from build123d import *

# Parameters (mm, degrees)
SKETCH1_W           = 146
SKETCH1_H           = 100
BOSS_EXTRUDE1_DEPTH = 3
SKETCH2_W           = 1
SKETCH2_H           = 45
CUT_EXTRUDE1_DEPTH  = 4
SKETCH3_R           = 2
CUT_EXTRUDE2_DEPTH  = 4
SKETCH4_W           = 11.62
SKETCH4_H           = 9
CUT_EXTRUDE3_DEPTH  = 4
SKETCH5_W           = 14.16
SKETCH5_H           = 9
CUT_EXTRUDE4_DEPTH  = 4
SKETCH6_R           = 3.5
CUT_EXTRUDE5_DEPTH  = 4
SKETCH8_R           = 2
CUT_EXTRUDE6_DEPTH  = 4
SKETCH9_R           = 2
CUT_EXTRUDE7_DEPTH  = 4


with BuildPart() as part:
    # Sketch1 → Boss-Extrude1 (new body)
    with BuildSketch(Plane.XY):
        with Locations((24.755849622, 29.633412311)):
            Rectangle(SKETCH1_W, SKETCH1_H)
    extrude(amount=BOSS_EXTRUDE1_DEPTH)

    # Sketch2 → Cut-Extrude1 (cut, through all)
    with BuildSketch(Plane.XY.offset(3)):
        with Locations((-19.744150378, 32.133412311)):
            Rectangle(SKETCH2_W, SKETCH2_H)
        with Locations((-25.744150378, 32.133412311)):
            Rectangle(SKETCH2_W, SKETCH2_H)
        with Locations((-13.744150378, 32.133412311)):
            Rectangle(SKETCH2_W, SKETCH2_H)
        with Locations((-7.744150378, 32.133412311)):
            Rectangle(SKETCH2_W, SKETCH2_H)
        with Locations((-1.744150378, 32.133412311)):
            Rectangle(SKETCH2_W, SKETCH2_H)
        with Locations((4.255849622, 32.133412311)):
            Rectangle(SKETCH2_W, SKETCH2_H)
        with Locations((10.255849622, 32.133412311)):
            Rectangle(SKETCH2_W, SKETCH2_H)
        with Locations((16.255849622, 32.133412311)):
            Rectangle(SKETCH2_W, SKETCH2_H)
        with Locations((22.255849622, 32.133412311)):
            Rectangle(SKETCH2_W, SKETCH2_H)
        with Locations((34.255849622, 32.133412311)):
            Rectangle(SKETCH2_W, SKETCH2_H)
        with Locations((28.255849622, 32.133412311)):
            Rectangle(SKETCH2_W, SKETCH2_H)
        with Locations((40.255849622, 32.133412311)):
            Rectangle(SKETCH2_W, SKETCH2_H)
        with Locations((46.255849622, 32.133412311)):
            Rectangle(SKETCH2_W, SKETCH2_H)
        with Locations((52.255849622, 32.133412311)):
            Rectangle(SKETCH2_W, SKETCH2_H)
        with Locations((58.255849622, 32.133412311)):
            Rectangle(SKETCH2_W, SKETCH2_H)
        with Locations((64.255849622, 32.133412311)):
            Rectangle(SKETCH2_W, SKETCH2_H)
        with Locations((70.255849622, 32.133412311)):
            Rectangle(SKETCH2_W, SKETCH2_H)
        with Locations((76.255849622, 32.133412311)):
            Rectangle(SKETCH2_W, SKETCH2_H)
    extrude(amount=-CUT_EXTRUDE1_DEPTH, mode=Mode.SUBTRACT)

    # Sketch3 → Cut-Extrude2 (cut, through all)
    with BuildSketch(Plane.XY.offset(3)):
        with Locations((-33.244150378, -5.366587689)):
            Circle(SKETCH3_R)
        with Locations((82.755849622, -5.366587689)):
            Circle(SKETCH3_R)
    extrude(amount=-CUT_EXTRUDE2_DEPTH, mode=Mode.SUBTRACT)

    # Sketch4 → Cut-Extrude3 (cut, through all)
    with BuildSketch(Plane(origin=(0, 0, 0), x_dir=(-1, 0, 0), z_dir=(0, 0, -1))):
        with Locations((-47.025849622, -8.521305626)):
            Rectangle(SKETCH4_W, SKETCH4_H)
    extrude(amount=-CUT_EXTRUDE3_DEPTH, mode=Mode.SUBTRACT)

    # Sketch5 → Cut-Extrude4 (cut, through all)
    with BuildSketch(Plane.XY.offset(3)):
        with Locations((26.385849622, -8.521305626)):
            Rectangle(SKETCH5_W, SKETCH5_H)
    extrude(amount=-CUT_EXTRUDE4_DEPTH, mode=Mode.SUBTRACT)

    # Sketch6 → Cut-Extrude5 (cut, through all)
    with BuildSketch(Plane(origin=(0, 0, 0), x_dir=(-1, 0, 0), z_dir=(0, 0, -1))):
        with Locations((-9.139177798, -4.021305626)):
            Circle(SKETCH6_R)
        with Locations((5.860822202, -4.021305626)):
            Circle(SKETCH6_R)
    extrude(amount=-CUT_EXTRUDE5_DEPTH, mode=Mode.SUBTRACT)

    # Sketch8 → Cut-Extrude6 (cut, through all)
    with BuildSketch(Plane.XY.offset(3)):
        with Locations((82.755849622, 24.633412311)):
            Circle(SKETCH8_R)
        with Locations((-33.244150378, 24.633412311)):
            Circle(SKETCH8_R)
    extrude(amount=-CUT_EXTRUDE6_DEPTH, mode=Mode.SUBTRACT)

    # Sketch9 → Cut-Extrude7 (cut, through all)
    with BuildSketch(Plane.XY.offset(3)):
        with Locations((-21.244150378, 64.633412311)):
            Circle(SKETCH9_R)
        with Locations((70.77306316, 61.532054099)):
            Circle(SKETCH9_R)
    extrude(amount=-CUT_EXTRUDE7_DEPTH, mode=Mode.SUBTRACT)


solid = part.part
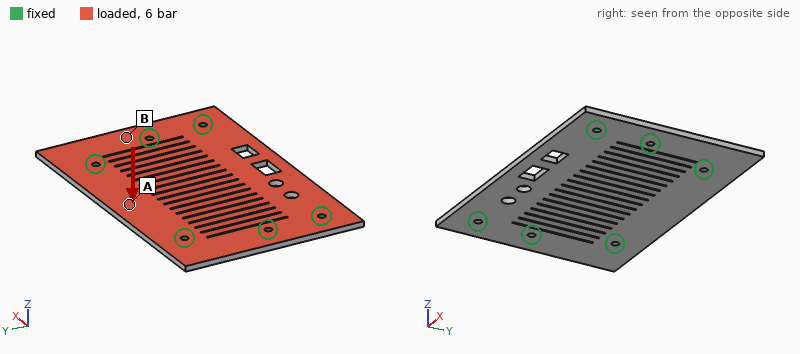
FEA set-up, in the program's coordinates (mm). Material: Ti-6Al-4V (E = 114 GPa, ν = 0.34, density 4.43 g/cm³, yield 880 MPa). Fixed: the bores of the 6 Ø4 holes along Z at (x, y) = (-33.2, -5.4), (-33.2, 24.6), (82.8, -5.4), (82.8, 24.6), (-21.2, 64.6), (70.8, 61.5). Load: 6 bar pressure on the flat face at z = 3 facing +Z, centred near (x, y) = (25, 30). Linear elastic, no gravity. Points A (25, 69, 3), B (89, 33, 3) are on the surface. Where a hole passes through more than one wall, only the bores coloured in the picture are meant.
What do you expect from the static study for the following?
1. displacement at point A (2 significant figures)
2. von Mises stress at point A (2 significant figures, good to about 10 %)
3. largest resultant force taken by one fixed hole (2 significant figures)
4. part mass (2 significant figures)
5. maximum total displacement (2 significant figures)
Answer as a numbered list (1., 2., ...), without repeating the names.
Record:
1. 0.76 mm
2. 250 MPa
3. 1.9 kN
4. 180 g
5. 1.6 mm
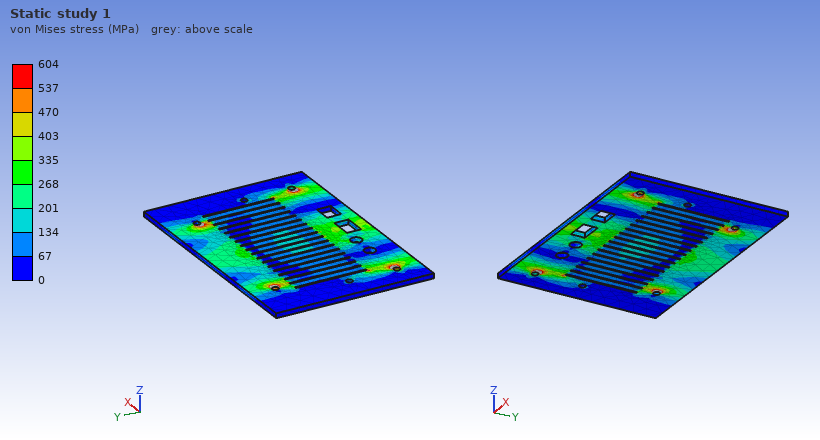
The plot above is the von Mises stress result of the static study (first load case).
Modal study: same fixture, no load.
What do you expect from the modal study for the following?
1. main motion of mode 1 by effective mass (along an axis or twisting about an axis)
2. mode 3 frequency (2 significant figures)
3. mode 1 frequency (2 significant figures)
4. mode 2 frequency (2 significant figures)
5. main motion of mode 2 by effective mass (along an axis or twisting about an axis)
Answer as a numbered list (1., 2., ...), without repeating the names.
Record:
1. along Z
2. 2300 Hz
3. 1000 Hz
4. 1700 Hz
5. twisting about X
